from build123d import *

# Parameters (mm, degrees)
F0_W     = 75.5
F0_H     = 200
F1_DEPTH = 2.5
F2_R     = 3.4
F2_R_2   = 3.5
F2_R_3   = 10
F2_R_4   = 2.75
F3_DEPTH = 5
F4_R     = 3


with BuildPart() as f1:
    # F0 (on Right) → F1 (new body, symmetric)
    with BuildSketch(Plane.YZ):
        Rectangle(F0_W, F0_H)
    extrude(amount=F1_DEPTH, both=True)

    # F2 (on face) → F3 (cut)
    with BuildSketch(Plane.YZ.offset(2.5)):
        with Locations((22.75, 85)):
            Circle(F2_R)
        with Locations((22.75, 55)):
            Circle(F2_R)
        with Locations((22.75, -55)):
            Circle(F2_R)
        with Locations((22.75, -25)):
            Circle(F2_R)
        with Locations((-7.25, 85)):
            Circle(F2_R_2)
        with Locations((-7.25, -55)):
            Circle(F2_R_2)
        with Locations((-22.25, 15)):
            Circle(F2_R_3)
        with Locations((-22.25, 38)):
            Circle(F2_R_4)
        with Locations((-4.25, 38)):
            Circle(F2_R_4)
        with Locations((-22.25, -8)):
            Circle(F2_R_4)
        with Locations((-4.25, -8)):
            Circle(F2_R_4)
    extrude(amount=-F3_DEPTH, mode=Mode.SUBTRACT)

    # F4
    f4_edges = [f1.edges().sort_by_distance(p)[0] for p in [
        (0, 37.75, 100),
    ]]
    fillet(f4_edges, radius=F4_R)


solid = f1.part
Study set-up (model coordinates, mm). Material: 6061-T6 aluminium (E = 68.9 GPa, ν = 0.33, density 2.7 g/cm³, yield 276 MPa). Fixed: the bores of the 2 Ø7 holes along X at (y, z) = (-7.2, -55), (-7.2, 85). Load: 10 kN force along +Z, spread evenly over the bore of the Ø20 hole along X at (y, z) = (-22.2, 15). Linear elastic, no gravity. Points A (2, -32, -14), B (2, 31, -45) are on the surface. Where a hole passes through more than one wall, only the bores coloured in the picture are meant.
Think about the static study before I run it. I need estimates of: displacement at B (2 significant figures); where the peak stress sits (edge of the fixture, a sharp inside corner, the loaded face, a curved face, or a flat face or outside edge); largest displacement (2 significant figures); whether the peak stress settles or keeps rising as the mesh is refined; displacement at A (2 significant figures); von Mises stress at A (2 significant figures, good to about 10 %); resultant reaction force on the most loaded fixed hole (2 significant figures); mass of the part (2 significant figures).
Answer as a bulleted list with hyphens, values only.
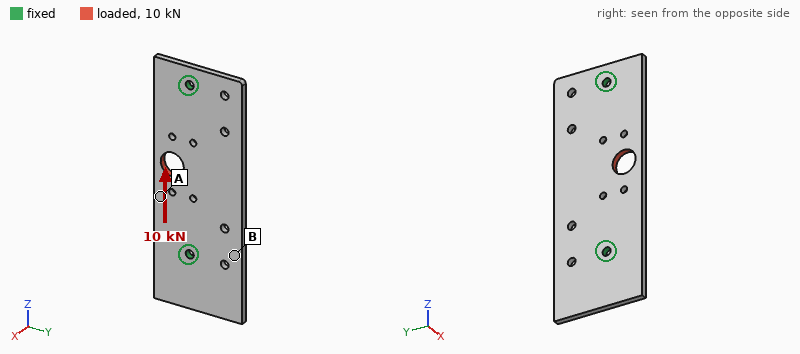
- 10.0 µm
- edge of the fixture
- 36 µm
- keeps rising
- 21 µm
- 31 MPa
- 5.3 kN
- 200 g
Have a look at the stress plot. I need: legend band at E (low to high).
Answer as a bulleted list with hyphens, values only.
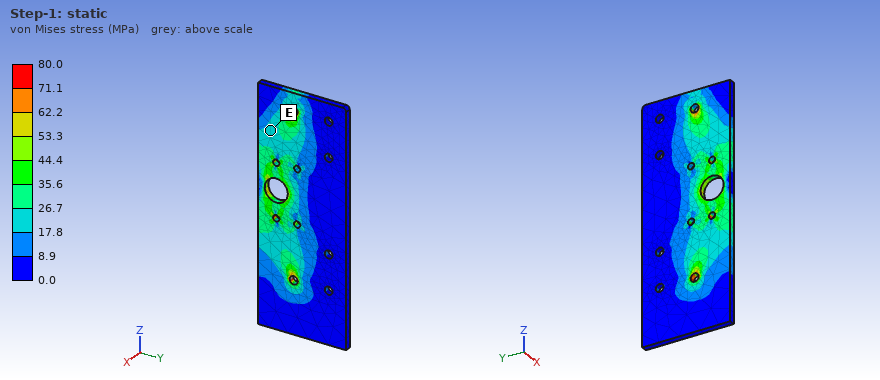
- 17.8 to 26.7 MPa
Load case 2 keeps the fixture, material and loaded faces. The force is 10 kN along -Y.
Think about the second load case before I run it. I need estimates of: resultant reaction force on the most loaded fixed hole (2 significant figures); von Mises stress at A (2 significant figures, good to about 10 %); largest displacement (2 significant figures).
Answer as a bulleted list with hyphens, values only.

- 5.2 kN
- 25 MPa
- 0.11 mm
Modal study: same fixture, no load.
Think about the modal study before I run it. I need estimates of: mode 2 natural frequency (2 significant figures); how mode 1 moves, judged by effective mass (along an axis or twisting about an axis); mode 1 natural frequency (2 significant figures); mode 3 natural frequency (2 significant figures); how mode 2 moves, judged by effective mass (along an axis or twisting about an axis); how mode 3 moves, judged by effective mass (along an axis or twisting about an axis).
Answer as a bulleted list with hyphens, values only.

- 1400 Hz
- along X
- 1000 Hz
- 1600 Hz
- twisting about Z
- along X
